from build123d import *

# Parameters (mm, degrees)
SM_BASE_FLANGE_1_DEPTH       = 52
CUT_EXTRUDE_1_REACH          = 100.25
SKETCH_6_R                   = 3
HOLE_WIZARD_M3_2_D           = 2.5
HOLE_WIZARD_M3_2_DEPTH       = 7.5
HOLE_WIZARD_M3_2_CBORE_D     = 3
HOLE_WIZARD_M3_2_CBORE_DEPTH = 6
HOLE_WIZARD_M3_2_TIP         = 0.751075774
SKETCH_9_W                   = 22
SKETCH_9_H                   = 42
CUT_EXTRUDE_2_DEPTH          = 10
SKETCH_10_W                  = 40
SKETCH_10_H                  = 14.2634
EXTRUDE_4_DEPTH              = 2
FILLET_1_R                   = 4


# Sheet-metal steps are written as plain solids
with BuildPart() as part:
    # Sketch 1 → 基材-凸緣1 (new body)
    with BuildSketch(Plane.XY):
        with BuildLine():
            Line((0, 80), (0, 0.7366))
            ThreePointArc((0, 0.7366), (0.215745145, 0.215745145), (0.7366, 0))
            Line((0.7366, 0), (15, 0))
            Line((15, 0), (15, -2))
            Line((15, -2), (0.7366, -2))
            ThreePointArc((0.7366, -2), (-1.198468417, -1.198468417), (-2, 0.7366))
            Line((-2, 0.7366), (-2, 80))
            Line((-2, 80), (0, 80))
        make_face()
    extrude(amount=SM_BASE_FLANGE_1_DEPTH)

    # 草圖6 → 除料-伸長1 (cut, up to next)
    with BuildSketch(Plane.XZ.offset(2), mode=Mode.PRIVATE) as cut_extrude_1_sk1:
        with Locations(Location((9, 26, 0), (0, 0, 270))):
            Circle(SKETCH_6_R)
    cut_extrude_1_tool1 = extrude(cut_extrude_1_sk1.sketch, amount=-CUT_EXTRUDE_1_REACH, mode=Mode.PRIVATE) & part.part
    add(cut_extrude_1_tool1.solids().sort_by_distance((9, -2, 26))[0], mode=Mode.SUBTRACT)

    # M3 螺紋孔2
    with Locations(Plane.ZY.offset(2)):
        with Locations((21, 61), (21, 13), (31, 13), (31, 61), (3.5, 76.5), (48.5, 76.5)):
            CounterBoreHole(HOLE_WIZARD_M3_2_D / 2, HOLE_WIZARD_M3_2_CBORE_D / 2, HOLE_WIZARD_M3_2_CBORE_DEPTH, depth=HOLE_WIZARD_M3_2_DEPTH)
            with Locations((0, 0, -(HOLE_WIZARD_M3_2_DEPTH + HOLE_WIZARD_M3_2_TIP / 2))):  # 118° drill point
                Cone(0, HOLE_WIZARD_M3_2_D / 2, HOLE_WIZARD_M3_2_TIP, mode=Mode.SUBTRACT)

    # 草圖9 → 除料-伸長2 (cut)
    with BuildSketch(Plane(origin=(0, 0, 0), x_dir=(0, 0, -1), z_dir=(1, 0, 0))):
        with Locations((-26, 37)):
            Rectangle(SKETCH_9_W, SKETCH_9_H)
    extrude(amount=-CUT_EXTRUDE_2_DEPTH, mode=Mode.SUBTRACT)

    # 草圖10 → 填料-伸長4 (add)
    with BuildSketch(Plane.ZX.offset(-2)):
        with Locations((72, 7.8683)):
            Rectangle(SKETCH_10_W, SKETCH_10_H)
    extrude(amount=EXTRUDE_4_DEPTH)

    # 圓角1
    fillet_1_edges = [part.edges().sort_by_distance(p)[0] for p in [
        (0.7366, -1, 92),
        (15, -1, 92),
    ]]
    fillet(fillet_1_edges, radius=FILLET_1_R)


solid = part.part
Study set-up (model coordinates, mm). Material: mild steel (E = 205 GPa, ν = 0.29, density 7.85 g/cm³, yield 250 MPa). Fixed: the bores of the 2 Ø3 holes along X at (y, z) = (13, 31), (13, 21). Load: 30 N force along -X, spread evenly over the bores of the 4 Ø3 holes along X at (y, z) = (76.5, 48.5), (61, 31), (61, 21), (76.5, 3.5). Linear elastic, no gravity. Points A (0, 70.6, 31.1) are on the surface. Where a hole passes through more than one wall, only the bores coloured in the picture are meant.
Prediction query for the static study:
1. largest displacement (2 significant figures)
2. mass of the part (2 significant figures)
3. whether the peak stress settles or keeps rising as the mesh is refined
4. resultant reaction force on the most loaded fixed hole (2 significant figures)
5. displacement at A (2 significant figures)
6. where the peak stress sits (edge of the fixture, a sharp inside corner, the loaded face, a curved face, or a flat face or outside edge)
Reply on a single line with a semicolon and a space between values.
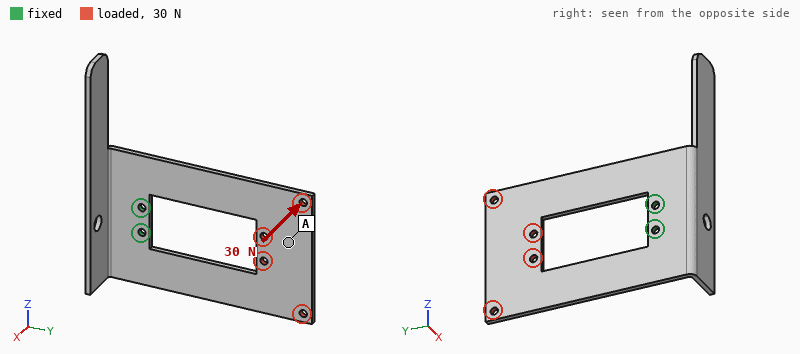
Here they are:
0.74 mm; 72 g; keeps rising; 15 N; 0.61 mm; edge of the fixture
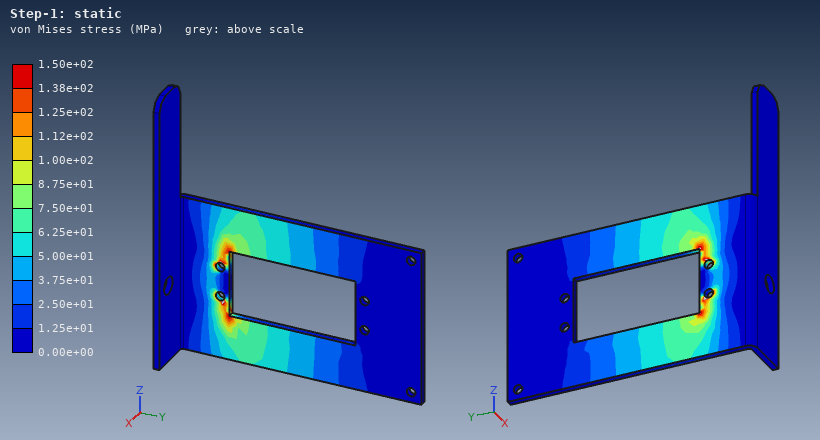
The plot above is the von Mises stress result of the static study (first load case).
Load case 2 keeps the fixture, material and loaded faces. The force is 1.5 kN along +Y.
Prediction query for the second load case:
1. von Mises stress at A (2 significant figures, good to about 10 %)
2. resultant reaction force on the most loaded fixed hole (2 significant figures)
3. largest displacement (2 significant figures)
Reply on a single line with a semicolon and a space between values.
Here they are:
14 MPa; 890 N; 23 µm
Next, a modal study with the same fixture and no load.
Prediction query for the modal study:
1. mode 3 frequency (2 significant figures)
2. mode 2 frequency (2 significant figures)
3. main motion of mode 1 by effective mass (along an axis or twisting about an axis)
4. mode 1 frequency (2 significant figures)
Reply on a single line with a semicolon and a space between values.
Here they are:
740 Hz; 720 Hz; along X; 250 Hz
